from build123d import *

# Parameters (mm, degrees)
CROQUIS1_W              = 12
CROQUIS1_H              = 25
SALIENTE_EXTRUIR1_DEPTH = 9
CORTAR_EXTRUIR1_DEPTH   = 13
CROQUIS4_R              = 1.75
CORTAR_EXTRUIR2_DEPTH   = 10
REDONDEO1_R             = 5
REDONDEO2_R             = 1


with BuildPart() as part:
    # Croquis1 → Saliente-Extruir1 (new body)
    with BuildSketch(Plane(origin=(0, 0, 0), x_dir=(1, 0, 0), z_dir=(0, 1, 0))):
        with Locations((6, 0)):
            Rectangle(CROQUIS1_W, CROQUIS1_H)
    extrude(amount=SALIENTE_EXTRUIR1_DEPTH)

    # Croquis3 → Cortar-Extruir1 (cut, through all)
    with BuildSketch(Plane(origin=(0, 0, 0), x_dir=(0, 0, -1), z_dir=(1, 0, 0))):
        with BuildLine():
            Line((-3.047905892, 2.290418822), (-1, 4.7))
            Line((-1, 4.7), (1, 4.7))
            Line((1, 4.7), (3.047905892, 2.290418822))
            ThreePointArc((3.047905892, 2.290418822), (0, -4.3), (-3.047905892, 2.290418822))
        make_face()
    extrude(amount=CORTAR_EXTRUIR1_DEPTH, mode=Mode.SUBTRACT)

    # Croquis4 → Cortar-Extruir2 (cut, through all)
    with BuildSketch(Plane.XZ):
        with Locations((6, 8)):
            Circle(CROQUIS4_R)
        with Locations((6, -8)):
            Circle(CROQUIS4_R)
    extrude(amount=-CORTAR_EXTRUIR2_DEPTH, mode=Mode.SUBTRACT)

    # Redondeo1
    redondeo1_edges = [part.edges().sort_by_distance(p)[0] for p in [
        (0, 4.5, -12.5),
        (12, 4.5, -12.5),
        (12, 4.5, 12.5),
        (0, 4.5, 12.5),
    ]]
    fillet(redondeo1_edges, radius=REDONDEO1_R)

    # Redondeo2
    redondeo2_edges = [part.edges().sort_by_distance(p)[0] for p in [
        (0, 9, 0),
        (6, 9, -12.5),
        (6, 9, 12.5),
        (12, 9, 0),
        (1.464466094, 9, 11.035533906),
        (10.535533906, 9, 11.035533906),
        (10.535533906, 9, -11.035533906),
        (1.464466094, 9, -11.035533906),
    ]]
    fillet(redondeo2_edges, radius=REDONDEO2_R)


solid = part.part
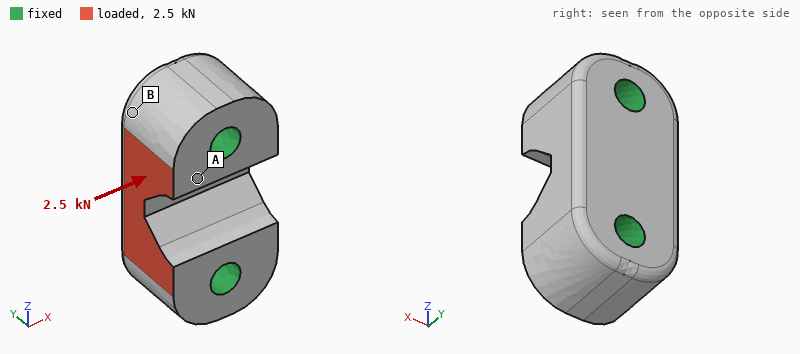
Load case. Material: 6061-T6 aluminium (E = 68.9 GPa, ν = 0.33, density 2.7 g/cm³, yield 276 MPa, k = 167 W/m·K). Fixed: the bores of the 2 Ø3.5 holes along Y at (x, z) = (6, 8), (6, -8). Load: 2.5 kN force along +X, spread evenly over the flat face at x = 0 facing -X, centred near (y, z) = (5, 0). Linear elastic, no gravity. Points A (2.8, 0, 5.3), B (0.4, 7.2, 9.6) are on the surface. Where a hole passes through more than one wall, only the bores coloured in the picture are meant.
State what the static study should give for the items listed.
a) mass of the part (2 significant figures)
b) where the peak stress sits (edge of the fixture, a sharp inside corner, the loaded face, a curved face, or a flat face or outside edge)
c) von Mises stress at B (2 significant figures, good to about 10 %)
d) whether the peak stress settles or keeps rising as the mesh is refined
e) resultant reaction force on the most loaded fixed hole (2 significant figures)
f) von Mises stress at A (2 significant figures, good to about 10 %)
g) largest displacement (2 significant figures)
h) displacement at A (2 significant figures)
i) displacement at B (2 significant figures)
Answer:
5.4 g
edge of the fixture
6.9 MPa
keeps rising
1.3 kN
27 MPa
4.3 µm
2.0 µm
0.92 µm
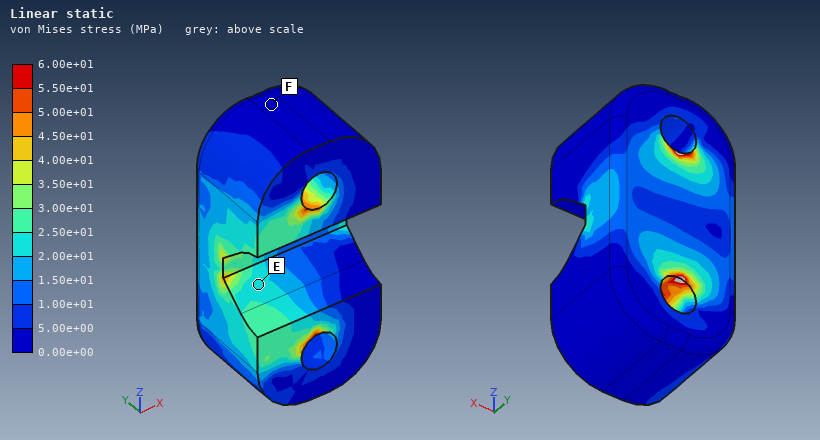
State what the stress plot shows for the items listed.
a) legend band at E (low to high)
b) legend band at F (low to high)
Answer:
2.00e+01 to 2.50e+01 MPa
0.00e+00 to 5.00e+00 MPa
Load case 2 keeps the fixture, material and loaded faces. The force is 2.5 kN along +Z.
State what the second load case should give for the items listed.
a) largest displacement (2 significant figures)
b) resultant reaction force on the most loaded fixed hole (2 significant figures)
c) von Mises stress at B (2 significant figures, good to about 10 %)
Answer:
6.9 µm
1.4 kN
14 MPa
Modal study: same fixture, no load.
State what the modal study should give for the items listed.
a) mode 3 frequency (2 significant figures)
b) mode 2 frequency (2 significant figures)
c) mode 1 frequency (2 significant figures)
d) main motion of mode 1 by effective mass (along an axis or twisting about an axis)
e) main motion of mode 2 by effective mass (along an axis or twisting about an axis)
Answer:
100 kHz
90 kHz
81 kHz
along X
along Y
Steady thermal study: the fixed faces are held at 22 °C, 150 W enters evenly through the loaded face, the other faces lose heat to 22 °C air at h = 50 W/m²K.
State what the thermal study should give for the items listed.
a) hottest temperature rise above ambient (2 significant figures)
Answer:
50 K
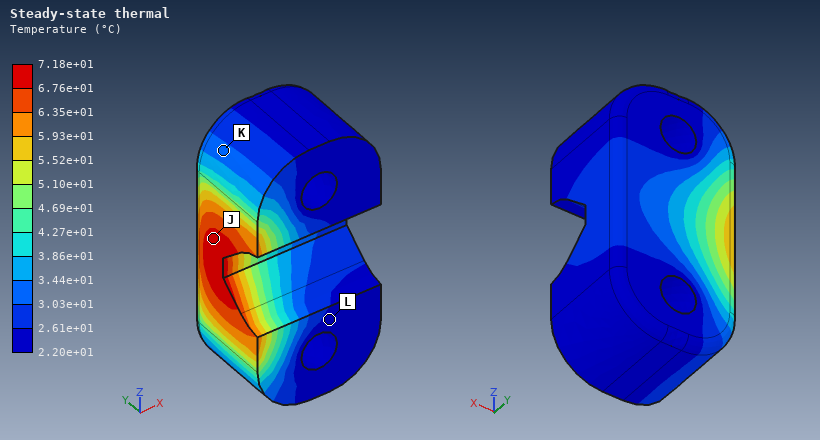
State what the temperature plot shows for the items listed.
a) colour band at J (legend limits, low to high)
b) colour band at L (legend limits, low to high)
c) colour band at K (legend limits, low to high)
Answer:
6.76e+01 to 7.18e+01 °C
2.20e+01 to 2.61e+01 °C
3.03e+01 to 3.44e+01 °C
